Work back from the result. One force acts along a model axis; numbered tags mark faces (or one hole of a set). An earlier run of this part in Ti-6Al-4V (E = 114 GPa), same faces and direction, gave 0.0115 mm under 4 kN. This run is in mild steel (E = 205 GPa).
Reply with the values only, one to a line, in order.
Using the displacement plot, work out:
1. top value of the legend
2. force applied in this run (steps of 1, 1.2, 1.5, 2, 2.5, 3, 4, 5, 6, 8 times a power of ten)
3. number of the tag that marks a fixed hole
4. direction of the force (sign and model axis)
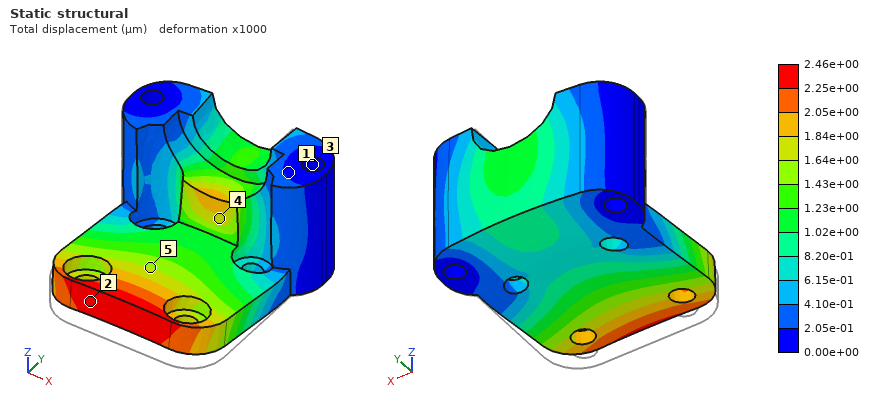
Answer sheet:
2.46e+00 µm
1.5 kN
3
+Y
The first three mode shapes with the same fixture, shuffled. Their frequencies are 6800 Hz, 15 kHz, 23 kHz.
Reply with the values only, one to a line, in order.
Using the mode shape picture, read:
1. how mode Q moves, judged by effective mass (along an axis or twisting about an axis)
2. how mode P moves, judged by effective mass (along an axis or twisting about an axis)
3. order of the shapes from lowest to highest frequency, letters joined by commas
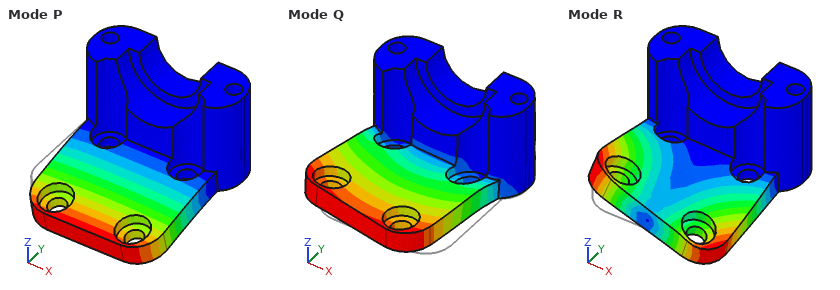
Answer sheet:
along X
along Z
P, R, Q
